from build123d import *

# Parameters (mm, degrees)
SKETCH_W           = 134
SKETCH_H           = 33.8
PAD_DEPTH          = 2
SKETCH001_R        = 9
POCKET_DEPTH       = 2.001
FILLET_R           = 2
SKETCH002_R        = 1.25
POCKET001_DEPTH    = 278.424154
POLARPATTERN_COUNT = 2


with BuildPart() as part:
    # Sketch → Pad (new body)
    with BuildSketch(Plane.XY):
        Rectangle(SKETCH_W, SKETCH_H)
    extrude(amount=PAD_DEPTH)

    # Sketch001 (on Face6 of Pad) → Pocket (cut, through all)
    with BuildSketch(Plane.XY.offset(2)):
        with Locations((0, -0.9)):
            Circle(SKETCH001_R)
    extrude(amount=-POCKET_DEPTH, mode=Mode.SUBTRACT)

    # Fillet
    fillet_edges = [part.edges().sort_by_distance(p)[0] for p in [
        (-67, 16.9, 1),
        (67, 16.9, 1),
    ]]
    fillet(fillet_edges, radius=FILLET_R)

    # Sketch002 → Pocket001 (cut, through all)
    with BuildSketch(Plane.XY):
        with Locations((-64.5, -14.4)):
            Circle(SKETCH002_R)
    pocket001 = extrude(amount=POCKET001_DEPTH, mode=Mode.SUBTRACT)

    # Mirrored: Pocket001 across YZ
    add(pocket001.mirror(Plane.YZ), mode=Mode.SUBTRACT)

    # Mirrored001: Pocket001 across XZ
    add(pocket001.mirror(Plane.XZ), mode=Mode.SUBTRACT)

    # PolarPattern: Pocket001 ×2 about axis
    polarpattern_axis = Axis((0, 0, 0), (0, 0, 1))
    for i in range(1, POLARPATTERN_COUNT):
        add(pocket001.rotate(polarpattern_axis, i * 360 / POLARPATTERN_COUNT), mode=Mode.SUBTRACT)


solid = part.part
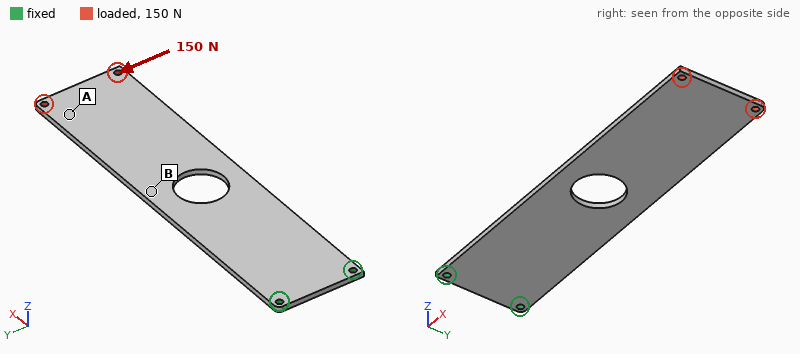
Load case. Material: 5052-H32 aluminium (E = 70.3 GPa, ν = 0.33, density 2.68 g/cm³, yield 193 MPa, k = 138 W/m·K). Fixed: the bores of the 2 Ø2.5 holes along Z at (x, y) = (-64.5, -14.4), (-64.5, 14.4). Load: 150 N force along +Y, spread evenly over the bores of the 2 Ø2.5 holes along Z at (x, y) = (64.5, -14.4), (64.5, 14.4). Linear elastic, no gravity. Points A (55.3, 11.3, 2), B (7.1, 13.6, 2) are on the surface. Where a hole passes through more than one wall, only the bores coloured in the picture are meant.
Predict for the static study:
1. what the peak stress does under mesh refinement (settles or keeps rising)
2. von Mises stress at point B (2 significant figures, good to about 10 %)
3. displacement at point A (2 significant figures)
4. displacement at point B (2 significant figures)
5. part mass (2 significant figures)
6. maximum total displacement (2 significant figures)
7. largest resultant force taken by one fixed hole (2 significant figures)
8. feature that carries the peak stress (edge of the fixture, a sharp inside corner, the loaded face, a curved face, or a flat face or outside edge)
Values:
keeps rising
16 MPa
0.25 mm
0.11 mm
23 g
0.28 mm
680 N
edge of the fixture
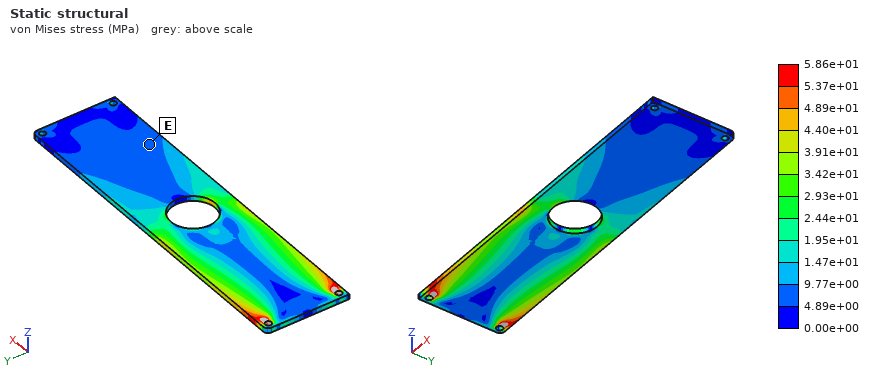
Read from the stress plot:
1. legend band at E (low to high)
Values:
4.89e+00 to 9.77e+00 MPa
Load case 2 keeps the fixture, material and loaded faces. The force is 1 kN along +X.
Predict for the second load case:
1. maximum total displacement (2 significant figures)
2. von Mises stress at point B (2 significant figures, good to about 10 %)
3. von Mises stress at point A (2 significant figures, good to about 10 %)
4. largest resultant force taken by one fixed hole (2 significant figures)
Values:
46 µm
25 MPa
22 MPa
520 N
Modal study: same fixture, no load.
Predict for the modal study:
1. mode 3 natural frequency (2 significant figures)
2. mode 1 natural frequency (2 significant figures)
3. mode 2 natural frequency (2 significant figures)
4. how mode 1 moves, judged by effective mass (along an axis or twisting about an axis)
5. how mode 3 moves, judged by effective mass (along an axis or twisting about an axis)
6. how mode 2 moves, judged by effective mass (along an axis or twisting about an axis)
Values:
710 Hz
90 Hz
550 Hz
along Z
twisting about X
along Z
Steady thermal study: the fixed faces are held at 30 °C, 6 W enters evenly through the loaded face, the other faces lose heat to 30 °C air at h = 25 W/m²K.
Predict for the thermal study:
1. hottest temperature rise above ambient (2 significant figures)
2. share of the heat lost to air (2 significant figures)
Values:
52 K
73 %
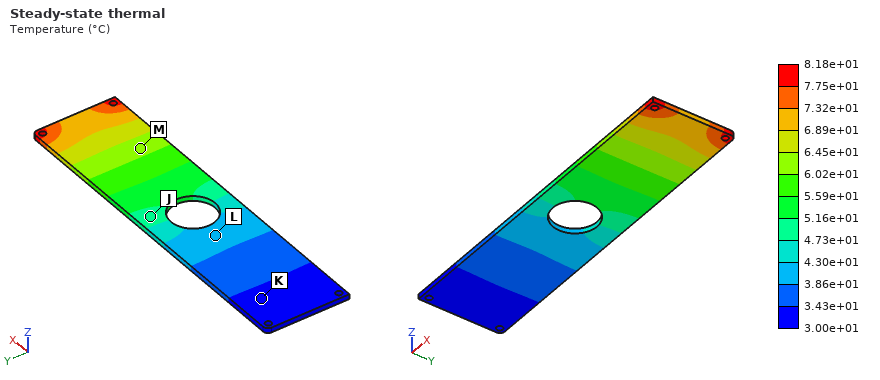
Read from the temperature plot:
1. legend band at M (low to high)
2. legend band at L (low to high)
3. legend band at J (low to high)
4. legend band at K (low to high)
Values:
6.02e+01 to 6.45e+01 °C
3.86e+01 to 4.30e+01 °C
4.73e+01 to 5.16e+01 °C
3.00e+01 to 3.43e+01 °C
